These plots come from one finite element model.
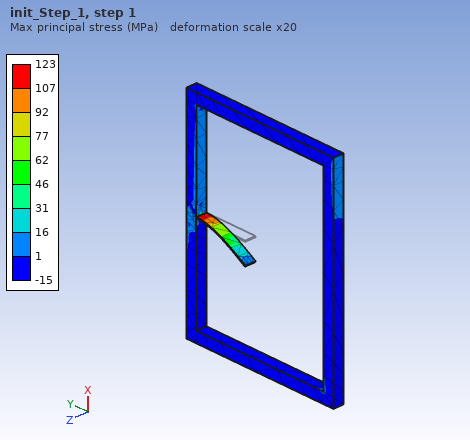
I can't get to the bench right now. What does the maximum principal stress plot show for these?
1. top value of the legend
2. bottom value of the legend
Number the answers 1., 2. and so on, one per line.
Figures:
1. 123 MPa
2. -15 MPa
